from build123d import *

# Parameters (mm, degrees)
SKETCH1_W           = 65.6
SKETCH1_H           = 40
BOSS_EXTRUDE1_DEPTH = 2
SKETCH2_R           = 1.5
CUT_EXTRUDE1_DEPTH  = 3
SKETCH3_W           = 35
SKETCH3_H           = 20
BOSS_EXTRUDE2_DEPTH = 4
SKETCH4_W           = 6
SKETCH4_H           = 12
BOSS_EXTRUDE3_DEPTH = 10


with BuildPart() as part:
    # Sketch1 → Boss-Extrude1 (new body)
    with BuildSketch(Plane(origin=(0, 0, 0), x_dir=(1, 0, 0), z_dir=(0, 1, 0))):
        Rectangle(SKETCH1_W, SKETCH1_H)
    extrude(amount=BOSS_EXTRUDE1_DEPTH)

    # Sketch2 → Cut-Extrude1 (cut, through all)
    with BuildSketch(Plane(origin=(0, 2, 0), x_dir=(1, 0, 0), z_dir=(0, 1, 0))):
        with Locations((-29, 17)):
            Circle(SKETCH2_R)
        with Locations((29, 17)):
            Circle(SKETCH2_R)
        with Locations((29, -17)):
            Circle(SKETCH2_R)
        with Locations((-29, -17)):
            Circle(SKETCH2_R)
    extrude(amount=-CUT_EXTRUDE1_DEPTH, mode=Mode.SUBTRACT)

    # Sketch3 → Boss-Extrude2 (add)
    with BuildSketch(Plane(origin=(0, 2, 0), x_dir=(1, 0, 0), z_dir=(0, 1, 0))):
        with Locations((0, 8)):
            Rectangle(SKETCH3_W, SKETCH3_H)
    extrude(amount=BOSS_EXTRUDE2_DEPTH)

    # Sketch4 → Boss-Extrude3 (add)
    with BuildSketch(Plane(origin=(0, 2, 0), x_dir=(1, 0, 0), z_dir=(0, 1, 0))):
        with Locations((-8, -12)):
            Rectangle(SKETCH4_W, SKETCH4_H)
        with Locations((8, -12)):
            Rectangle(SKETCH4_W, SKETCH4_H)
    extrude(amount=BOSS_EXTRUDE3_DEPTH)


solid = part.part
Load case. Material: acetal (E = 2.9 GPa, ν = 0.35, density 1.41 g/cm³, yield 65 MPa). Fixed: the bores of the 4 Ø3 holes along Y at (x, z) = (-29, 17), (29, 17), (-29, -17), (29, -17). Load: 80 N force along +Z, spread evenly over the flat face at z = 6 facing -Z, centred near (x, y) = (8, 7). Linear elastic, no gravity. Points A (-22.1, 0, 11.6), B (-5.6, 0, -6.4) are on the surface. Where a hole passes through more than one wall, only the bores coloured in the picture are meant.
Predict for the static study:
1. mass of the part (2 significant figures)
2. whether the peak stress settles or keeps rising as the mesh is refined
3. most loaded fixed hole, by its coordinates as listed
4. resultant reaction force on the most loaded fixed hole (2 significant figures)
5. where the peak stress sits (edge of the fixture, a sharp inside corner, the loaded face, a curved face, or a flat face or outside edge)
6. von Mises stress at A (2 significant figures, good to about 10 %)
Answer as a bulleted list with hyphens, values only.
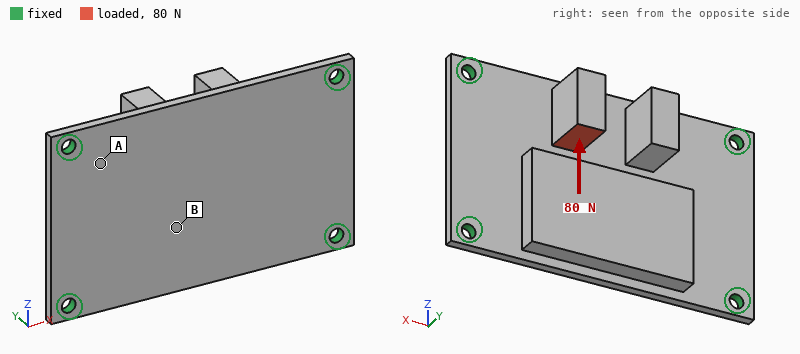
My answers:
- 13 g
- keeps rising
- (29, -17)
- 36 N
- edge of the fixture
- 3.0 MPa
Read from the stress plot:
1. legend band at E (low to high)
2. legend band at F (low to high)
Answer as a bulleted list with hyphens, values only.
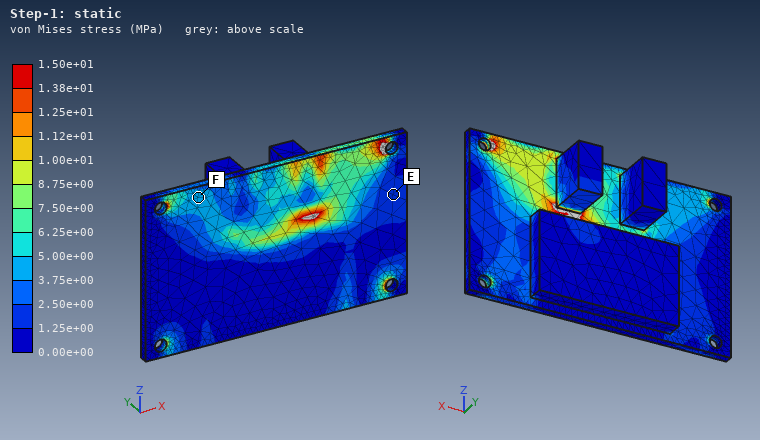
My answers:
- 1.25e+00 to 2.50e+00 MPa
- 3.75e+00 to 5.00e+00 MPa
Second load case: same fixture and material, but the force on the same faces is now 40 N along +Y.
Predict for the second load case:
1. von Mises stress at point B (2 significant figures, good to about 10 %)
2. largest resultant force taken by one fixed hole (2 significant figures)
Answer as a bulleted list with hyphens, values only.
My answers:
- 1.7 MPa
- 19 N
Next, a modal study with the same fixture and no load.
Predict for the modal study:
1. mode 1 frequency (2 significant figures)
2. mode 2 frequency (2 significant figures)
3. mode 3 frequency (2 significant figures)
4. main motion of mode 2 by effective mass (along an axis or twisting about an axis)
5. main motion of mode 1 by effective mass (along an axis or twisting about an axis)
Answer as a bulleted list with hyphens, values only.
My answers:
- 770 Hz
- 1200 Hz
- 1900 Hz
- along Y
- along Y
